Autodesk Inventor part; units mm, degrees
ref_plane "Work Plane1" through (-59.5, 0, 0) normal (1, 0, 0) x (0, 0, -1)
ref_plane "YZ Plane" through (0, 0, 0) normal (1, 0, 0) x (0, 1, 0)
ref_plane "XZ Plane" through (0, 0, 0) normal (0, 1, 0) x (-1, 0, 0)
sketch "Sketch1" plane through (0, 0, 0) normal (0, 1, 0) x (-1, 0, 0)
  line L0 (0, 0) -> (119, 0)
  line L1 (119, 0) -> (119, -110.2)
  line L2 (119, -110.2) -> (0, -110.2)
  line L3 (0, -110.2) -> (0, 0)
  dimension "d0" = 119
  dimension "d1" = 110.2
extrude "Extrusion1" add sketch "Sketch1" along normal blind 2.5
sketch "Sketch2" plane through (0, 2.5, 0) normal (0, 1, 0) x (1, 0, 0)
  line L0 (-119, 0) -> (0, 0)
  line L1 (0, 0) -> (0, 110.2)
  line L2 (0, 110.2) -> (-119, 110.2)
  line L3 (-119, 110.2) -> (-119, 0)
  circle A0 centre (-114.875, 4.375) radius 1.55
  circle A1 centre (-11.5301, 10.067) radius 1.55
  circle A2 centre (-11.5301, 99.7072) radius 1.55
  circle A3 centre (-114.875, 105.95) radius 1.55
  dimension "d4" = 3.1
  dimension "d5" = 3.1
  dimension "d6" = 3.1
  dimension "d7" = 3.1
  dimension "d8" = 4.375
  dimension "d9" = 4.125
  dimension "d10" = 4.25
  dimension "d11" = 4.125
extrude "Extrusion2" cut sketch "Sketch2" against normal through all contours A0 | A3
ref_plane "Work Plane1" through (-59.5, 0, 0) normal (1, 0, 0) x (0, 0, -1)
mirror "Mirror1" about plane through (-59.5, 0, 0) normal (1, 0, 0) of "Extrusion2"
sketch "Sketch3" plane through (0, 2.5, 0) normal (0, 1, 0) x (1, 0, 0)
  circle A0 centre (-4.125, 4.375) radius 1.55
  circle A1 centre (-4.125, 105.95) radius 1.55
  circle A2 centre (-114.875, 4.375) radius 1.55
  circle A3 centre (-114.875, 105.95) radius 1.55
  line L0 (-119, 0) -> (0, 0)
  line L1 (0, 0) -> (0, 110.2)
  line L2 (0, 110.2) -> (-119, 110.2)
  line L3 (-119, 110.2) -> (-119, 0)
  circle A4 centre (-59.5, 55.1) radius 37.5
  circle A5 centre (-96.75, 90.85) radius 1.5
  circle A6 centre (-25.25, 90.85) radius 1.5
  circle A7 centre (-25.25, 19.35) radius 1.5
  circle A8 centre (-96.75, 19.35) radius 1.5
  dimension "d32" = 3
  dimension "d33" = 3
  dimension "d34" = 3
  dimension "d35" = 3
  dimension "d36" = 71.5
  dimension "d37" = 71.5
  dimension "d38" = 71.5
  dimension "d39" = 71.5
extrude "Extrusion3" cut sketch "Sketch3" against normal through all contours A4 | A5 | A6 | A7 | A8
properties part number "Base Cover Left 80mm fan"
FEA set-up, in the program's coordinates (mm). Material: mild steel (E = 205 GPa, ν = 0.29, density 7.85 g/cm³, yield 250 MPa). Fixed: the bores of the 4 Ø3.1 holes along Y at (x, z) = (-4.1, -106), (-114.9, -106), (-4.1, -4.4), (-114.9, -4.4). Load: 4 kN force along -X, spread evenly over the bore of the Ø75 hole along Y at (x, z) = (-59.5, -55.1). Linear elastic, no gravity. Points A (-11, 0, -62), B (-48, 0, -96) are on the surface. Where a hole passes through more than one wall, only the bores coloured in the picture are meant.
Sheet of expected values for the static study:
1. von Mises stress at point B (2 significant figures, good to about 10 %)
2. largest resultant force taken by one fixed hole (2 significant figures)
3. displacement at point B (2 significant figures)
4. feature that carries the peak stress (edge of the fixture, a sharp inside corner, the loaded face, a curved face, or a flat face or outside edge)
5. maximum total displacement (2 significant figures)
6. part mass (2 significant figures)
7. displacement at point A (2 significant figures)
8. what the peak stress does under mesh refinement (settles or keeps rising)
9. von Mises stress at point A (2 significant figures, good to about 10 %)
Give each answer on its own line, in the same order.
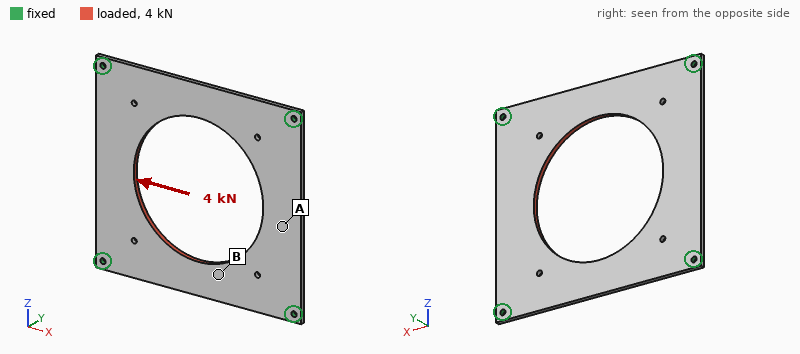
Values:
18 MPa
1.1 kN
5.2 µm
edge of the fixture
11 µm
170 g
11 µm
keeps rising
7.4 MPa
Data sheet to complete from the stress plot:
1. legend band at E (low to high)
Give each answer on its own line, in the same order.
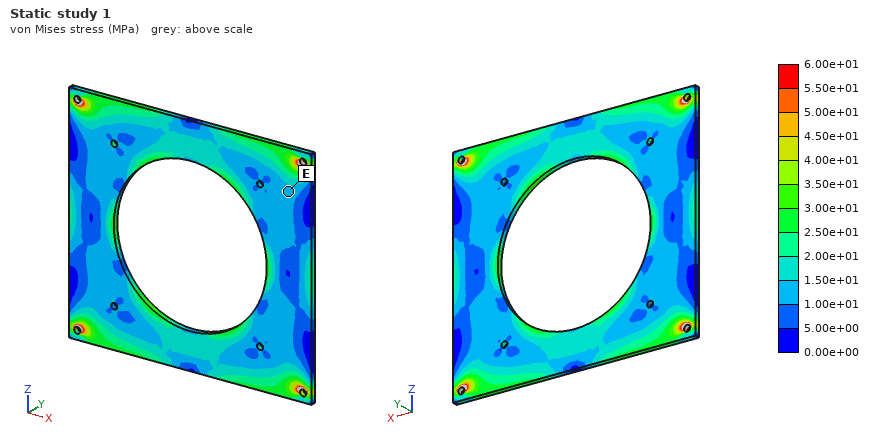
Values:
1.00e+01 to 1.50e+01 MPa
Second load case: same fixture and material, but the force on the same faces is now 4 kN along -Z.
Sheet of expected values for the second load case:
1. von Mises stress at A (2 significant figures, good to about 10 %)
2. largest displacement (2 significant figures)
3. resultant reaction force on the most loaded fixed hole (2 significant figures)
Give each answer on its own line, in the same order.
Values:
20 MPa
14 µm
1.1 kN
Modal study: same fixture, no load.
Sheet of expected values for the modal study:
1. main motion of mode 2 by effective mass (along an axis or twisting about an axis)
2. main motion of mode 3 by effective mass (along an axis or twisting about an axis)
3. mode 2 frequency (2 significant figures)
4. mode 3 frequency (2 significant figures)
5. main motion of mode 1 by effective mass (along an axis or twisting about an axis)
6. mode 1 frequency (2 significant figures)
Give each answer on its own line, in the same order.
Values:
twisting about X
twisting about Z
1100 Hz
1200 Hz
along Y
870 Hz
